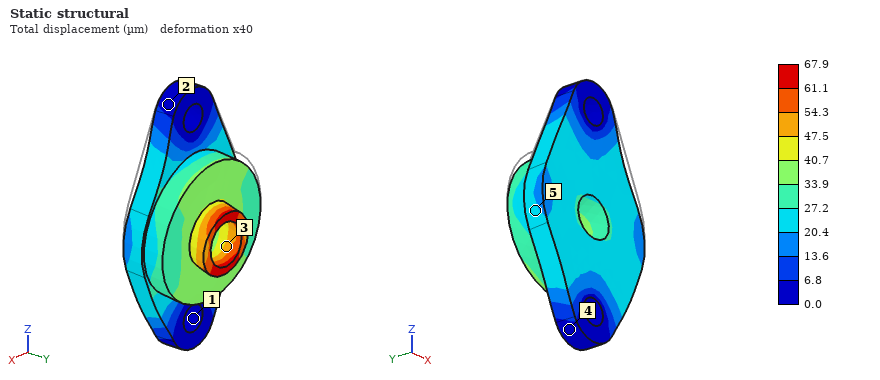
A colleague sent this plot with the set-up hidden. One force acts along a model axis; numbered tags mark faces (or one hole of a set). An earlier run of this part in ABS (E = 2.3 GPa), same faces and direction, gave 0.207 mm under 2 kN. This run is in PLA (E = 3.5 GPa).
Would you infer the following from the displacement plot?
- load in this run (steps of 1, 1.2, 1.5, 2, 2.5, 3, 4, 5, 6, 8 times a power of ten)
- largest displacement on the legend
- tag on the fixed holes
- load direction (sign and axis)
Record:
1 kN
67.9 µm
1
-Z
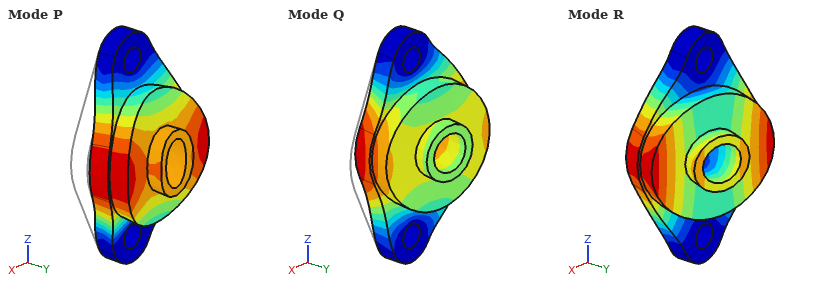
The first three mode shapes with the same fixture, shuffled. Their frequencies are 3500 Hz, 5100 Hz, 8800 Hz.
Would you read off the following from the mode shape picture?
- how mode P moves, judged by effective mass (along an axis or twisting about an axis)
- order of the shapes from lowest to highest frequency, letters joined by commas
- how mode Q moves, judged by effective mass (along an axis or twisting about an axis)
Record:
along Y
R, P, Q
along X
